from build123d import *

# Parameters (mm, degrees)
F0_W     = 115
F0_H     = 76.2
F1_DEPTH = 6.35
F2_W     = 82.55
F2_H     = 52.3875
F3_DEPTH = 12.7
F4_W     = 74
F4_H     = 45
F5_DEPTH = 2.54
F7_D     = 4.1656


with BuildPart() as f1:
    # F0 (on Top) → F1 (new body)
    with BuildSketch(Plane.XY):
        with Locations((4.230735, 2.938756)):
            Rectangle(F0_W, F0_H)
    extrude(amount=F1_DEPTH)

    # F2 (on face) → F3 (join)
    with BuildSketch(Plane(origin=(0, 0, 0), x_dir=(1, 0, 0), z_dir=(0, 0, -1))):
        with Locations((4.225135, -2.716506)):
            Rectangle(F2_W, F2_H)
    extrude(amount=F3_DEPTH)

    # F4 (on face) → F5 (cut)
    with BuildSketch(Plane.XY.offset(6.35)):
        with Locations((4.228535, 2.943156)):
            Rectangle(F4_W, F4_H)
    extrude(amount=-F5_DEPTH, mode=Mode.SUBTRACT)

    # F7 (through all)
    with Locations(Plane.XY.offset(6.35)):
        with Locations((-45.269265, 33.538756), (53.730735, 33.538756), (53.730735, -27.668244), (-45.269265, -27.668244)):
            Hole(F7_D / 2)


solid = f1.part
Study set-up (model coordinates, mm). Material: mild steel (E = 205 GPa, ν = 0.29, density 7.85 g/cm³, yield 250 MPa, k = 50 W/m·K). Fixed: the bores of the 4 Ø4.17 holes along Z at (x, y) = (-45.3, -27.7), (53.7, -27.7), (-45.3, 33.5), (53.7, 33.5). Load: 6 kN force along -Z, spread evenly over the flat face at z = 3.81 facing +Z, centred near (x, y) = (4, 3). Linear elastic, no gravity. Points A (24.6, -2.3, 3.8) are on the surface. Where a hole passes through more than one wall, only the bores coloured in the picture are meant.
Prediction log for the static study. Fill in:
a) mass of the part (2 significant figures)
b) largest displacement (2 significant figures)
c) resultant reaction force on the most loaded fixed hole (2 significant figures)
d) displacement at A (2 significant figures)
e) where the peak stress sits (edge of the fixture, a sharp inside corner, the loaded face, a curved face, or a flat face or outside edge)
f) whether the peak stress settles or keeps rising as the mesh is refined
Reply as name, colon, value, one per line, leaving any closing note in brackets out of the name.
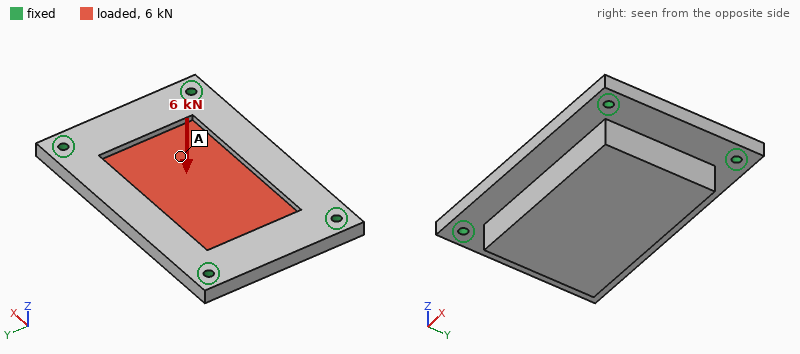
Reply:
mass of the part: 800 g
largest displacement: 17 µm
resultant reaction force on the most loaded fixed hole: 2.2 kN
displacement at A: 14 µm
where the peak stress sits: edge of the fixture
whether the peak stress settles or keeps rising as the mesh is refined: keeps rising
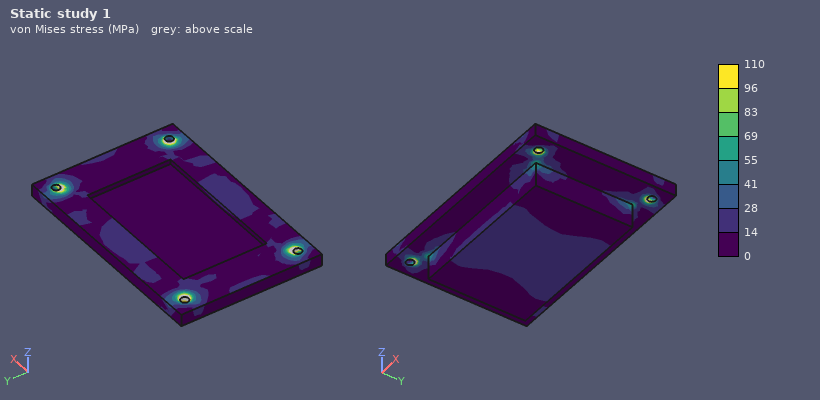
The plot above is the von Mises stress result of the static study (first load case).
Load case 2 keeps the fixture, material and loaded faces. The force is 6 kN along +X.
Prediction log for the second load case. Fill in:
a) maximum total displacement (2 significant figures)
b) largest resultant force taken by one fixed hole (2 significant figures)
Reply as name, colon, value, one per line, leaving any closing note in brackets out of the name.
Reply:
maximum total displacement: 2.3 µm
largest resultant force taken by one fixed hole: 1.6 kN
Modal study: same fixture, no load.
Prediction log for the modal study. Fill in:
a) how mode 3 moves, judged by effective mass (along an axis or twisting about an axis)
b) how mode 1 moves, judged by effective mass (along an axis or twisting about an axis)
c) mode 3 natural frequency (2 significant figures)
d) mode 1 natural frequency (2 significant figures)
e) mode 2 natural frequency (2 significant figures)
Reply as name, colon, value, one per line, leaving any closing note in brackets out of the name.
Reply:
how mode 3 moves, judged by effective mass: twisting about Y
how mode 1 moves, judged by effective mass: along Z
mode 3 natural frequency: 7900 Hz
mode 1 natural frequency: 4000 Hz
mode 2 natural frequency: 6000 Hz
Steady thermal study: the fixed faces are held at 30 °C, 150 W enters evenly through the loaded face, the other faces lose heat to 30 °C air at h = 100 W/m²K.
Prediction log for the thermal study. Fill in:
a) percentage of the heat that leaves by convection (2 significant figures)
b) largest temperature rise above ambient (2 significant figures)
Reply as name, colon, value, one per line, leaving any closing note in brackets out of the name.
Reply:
percentage of the heat that leaves by convection: 53 %
largest temperature rise above ambient: 68 K
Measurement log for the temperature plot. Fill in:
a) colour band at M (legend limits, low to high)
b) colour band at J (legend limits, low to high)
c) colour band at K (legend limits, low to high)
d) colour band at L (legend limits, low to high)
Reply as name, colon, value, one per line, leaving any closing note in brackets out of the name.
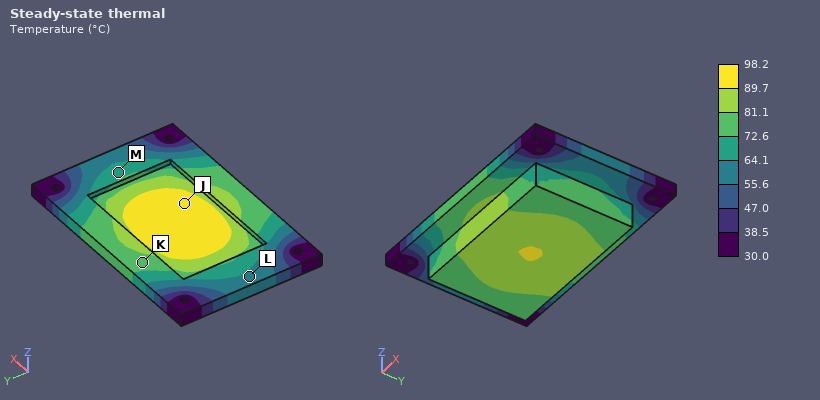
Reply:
colour band at M: 64.1 to 72.6 °C
colour band at J: 89.7 to 98.2 °C
colour band at K: 72.6 to 81.1 °C
colour band at L: 55.6 to 64.1 °C
